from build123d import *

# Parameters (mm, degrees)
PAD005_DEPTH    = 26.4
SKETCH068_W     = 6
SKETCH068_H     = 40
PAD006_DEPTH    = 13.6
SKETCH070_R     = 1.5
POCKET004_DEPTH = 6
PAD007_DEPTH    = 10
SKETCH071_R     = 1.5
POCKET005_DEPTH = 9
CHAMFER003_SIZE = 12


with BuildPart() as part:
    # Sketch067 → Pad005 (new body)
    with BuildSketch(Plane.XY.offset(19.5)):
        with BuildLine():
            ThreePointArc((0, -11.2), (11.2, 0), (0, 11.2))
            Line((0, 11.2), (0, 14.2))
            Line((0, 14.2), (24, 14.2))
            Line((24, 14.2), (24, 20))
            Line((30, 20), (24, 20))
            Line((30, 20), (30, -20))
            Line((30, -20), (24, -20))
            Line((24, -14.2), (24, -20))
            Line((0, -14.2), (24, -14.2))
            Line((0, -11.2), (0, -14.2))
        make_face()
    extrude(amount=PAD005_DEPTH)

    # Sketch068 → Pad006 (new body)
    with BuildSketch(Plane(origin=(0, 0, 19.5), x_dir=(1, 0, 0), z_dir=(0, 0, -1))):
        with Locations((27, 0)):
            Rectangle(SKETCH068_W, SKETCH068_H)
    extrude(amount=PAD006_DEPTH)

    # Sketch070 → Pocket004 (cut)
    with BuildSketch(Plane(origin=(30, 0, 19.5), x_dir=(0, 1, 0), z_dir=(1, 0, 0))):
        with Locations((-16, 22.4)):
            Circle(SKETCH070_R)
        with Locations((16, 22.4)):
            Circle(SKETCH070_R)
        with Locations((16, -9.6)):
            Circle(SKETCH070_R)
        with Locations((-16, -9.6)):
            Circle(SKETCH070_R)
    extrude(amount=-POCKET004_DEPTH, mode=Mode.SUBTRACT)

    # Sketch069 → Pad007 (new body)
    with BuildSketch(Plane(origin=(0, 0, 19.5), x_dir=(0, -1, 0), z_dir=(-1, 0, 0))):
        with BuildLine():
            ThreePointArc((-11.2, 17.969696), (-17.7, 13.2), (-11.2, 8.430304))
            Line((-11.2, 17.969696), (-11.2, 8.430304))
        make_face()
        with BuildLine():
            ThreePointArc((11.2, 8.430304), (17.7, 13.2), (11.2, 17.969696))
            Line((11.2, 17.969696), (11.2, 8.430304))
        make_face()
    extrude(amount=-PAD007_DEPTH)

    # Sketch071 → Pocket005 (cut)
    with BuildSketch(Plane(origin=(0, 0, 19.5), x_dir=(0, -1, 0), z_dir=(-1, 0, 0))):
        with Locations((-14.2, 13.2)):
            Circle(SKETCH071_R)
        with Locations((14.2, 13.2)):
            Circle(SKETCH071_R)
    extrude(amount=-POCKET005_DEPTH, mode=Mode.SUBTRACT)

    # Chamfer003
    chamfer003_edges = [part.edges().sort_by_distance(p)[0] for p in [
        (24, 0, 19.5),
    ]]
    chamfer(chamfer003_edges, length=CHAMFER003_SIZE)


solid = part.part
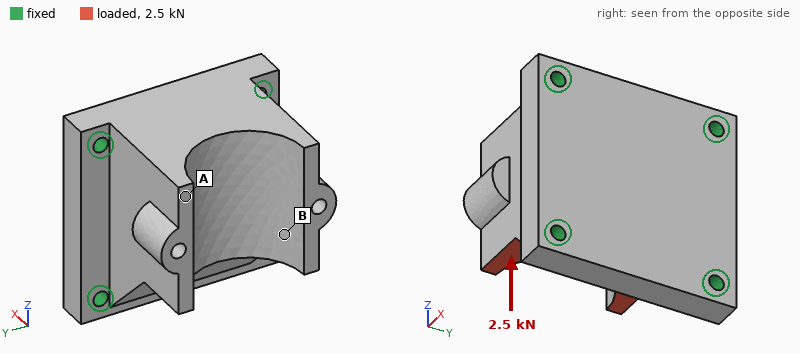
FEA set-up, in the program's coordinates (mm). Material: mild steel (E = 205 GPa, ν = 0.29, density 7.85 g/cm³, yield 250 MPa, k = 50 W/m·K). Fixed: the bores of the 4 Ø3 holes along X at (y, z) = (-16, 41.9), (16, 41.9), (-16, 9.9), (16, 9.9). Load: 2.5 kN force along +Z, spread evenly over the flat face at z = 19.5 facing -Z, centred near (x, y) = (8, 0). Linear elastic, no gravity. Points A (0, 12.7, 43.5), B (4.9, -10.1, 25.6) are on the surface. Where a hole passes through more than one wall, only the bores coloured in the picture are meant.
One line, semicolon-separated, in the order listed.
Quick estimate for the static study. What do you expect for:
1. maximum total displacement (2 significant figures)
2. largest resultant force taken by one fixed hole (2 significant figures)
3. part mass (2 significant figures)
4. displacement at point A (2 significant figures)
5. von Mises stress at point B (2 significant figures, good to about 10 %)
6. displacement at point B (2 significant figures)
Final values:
5.0 µm; 1.1 kN; 190 g; 3.8 µm; 15 MPa; 3.5 µm
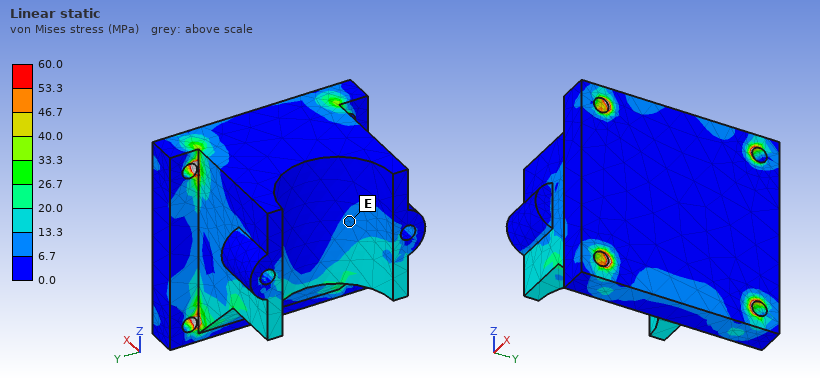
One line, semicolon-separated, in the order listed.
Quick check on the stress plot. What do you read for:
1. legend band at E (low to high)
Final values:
6.7 to 13.3 MPa
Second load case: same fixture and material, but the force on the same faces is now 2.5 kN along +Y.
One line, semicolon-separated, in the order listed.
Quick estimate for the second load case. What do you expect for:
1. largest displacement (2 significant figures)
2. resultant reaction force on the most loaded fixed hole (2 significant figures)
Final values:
15 µm; 1.1 kN
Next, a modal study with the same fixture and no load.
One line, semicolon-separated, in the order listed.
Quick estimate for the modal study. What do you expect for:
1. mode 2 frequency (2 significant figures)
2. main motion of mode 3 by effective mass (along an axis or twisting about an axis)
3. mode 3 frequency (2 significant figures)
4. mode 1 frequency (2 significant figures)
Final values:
17 kHz; along X; 18 kHz; 17 kHz
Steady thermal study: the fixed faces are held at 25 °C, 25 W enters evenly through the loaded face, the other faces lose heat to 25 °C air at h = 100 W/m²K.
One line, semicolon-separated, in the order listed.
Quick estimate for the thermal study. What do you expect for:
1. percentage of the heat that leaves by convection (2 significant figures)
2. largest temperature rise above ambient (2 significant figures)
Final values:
27 %; 42 K
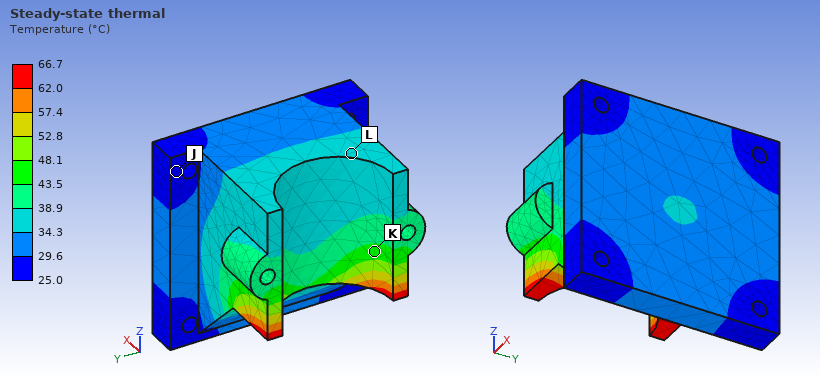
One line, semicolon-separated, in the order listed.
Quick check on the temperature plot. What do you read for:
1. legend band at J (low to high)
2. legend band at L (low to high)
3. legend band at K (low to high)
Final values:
25.0 to 29.6 °C; 34.3 to 38.9 °C; 43.5 to 48.1 °C
